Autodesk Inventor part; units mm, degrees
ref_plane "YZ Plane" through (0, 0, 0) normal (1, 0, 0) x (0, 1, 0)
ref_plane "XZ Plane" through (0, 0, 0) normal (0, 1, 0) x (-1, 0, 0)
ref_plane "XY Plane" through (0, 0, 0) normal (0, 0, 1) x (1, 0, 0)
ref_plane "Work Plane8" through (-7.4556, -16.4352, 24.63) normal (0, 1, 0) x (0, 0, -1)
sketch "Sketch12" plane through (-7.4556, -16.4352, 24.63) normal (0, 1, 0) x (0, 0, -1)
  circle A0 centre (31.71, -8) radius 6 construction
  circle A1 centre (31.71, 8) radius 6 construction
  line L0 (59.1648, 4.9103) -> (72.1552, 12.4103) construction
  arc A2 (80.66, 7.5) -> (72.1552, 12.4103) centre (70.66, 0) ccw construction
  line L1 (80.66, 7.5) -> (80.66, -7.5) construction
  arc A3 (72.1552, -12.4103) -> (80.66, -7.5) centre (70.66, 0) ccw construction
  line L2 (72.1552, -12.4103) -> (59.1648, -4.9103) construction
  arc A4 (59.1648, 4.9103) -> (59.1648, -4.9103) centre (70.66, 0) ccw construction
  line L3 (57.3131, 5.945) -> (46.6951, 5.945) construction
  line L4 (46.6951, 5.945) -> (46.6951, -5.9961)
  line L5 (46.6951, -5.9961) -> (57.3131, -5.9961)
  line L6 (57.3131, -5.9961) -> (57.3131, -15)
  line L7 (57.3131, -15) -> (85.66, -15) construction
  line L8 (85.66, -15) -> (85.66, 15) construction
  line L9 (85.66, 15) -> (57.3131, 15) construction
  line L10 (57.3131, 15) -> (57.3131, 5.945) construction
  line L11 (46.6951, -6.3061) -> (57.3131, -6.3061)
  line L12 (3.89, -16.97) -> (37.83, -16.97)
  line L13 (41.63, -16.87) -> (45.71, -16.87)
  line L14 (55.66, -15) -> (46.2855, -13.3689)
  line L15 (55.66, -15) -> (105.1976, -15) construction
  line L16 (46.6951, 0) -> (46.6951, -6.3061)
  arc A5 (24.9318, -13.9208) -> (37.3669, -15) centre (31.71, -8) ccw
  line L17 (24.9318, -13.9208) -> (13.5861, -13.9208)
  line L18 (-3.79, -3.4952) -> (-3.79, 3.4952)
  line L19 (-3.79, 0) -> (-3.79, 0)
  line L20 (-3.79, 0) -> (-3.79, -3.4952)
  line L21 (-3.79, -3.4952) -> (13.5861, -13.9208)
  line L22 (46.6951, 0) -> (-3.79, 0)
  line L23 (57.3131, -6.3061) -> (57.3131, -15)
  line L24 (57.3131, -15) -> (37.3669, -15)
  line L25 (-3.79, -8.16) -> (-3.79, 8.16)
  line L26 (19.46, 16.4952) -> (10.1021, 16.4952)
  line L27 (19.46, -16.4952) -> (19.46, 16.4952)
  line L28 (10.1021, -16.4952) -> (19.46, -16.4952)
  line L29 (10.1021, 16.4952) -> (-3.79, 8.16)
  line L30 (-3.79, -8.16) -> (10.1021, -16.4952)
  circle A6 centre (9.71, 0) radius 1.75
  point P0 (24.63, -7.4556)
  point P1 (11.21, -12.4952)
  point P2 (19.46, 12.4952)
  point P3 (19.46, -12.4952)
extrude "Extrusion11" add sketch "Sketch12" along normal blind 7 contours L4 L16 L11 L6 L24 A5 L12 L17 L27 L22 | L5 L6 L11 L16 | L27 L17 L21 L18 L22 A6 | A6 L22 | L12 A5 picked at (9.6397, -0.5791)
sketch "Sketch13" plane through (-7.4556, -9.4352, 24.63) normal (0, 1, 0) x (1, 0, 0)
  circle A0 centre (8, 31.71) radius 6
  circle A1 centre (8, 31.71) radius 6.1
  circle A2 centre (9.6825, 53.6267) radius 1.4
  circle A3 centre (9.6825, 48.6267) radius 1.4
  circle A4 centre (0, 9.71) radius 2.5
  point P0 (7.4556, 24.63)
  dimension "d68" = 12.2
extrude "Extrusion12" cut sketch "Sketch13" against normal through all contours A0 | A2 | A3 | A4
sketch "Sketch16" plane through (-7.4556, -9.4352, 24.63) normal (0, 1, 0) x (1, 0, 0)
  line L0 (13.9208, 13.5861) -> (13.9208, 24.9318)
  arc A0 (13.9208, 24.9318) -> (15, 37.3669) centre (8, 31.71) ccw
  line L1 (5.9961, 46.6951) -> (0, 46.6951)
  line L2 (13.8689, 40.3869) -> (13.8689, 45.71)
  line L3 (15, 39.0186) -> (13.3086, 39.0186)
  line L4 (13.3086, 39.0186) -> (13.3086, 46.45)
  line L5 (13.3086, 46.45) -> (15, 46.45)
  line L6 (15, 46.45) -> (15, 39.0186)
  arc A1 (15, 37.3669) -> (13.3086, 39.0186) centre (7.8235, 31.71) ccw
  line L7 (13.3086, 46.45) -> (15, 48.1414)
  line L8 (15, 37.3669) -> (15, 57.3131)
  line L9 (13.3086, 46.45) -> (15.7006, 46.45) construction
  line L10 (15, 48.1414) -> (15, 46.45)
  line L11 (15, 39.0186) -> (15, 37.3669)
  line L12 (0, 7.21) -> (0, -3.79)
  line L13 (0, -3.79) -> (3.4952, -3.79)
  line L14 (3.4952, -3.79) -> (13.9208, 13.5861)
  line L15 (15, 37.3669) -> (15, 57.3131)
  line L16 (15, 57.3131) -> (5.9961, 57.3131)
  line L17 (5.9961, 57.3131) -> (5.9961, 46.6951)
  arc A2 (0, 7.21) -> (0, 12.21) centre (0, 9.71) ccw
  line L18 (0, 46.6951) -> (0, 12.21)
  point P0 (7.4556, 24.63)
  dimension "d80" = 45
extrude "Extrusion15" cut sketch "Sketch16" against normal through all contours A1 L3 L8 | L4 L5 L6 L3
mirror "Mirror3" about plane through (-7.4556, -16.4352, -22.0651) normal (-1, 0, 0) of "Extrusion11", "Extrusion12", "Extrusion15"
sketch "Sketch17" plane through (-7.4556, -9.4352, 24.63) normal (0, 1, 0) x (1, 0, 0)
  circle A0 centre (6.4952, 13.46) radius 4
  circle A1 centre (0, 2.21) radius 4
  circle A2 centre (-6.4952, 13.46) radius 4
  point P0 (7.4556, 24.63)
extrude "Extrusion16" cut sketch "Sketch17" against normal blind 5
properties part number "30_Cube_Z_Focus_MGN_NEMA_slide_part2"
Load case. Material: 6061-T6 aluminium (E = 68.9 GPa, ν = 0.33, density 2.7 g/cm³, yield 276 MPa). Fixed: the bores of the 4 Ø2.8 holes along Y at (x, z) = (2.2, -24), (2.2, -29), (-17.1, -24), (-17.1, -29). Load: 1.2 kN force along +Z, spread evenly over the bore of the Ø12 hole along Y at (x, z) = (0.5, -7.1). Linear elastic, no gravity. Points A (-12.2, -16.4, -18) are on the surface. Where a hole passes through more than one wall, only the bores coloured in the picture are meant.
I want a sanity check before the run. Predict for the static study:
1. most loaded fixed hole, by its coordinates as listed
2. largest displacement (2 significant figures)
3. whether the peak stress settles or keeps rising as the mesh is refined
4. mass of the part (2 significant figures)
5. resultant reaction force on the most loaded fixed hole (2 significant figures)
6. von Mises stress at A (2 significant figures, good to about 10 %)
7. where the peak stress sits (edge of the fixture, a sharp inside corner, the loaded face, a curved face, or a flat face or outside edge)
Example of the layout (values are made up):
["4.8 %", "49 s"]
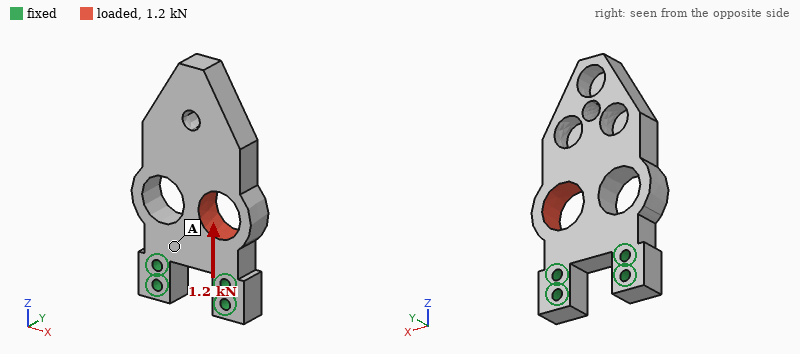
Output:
["(2.2, -24)", "24 µm", "keeps rising", "21 g", "940 N", "6.9 MPa", "a sharp inside corner"]
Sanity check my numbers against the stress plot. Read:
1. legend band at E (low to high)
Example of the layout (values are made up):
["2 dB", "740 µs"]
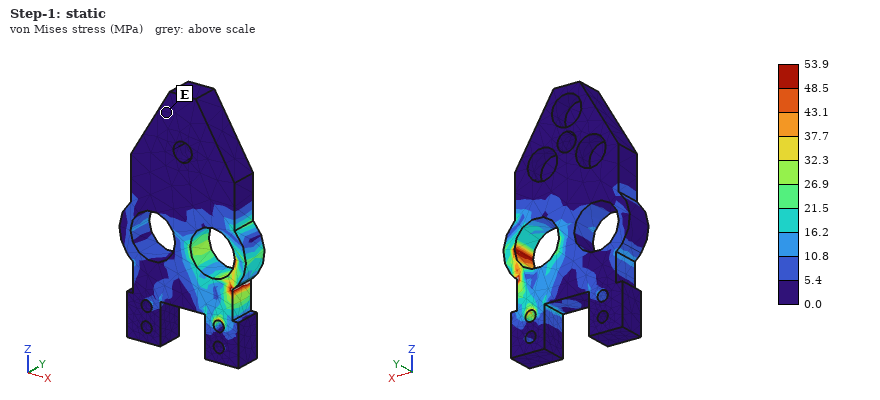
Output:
["0.0 to 5.4 MPa"]
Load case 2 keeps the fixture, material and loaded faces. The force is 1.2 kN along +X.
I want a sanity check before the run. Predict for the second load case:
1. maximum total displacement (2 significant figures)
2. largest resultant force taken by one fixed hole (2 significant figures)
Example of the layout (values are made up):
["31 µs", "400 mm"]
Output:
["45 µm", "1.0 kN"]
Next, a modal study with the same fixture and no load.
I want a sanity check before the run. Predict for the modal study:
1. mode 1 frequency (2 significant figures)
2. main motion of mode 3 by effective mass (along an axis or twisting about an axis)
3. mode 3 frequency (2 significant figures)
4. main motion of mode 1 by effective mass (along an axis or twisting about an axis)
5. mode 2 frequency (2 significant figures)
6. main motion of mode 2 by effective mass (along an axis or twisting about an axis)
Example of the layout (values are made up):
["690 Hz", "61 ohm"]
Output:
["2000 Hz", "twisting about Z", "8100 Hz", "along Y", "5600 Hz", "along X"]
